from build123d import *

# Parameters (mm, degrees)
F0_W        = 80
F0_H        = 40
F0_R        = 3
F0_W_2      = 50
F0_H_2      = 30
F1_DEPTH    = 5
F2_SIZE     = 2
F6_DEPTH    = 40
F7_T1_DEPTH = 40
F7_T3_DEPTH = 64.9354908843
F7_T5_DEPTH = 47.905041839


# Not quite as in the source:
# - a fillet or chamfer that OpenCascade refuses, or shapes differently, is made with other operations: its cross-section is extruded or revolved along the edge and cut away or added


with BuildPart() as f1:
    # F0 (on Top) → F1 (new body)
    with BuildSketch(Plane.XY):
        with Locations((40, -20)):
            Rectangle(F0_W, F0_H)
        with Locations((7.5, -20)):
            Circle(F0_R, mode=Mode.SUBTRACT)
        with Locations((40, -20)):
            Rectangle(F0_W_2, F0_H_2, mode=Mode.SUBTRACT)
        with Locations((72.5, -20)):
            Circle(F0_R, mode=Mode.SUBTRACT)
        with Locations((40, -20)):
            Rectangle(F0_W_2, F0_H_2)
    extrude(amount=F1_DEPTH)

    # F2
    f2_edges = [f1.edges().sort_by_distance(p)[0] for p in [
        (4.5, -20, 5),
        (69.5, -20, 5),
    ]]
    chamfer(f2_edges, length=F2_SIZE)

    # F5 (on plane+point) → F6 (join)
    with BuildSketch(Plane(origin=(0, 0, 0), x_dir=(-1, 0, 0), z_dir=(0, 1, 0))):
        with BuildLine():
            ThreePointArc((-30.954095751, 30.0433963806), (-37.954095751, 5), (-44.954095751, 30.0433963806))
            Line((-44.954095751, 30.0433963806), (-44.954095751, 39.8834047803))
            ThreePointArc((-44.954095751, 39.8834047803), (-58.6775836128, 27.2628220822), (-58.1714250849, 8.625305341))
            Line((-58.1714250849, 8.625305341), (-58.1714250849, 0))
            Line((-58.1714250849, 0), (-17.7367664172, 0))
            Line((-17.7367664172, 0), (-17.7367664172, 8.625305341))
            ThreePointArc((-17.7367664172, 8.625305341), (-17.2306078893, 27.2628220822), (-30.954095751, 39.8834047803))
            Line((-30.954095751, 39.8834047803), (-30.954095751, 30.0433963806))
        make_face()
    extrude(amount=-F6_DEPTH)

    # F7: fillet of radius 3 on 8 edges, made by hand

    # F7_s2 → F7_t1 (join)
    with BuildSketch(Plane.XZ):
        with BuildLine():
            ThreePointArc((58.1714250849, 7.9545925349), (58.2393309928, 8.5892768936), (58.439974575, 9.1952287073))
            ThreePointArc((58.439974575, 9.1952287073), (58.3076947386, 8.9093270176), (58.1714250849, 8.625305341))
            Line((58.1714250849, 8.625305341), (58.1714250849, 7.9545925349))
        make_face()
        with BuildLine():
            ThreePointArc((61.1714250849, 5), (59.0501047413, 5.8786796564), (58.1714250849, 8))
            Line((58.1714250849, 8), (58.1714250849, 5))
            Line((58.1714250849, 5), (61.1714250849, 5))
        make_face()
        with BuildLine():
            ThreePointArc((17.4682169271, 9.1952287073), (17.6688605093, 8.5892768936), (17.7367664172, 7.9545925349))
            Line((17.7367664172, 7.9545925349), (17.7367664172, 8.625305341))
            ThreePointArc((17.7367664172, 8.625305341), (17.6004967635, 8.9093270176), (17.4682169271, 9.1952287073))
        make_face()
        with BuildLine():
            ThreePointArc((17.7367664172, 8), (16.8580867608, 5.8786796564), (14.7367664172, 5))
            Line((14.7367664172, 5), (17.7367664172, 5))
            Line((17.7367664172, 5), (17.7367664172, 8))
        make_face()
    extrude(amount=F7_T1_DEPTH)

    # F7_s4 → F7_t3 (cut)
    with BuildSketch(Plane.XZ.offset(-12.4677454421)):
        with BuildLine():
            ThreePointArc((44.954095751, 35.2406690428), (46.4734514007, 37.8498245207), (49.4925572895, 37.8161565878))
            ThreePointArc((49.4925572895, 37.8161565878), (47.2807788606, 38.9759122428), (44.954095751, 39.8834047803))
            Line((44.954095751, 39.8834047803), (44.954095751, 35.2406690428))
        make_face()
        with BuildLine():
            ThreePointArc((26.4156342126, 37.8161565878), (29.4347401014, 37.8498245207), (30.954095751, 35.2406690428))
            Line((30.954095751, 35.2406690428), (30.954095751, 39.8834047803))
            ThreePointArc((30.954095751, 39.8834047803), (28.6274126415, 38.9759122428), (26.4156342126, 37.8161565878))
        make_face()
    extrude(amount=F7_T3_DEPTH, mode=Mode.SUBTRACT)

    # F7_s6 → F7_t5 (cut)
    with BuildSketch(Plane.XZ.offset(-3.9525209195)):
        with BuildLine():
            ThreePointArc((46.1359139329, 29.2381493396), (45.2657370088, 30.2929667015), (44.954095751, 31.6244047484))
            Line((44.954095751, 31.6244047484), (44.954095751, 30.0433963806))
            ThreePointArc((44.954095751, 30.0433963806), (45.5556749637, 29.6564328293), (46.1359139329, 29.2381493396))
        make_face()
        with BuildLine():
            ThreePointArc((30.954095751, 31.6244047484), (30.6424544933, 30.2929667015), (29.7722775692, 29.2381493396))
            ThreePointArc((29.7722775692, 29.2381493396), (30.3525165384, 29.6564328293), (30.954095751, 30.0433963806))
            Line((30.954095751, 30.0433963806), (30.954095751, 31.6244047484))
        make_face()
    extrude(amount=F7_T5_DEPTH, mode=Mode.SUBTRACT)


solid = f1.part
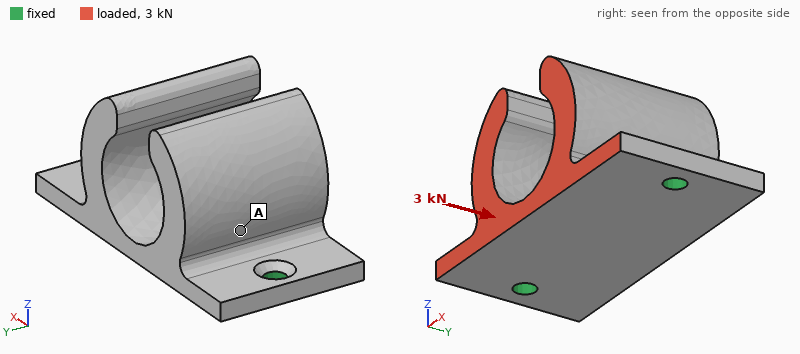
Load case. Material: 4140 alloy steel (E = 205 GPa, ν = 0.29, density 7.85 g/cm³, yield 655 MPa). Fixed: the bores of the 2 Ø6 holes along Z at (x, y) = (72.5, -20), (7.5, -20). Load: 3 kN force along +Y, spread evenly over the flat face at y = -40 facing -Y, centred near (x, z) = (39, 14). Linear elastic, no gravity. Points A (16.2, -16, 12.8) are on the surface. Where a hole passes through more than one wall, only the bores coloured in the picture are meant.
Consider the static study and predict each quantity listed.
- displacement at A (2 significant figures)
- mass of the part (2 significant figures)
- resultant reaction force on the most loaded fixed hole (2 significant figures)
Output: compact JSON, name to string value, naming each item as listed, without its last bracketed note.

{"displacement at A": "29 µm", "mass of the part": "330 g", "resultant reaction force on the most loaded fixed hole": "1.6 kN"}
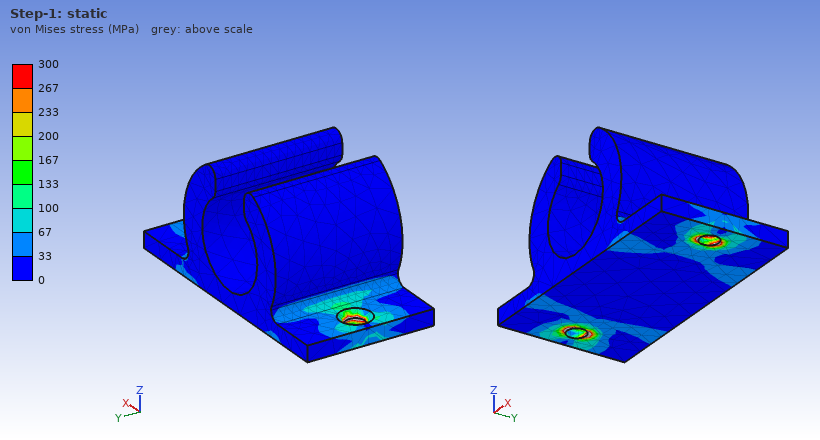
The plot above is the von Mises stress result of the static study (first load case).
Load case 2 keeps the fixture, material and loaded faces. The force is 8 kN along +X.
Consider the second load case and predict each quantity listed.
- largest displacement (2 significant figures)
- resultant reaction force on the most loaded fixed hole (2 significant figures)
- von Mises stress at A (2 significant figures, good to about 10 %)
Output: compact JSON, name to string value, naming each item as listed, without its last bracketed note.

{"largest displacement": "60 µm", "resultant reaction force on the most loaded fixed hole": "5.0 kN", "von Mises stress at A": "41 MPa"}
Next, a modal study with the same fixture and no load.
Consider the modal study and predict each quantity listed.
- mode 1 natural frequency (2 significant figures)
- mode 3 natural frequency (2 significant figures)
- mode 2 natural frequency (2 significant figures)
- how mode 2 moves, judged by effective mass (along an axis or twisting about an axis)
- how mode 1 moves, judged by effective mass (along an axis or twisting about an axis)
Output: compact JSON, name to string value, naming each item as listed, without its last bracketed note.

{"mode 1 natural frequency": "1700 Hz", "mode 3 natural frequency": "4300 Hz", "mode 2 natural frequency": "2400 Hz", "how mode 2 moves, judged by effective mass": "along Z", "how mode 1 moves, judged by effective mass": "along Y"}
